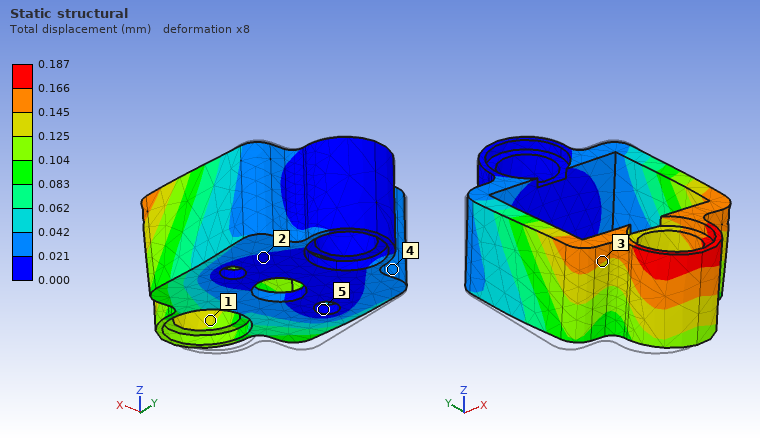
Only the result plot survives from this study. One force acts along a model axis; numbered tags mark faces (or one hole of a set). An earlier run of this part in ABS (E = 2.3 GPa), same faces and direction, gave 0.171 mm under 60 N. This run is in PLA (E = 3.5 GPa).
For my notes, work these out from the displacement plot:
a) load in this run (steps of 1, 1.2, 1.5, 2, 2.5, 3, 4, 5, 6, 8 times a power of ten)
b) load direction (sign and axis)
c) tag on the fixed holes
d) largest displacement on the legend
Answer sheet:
100 N
+X
5
0.187 mm
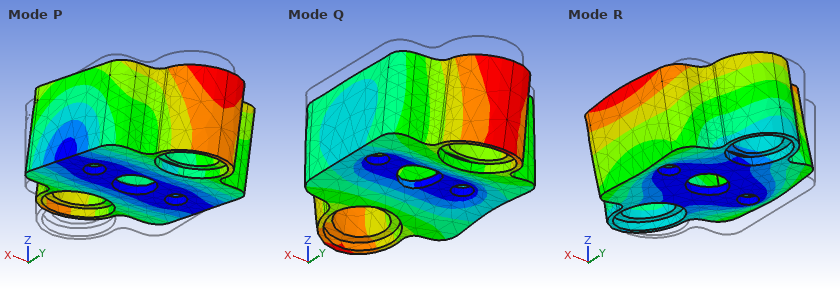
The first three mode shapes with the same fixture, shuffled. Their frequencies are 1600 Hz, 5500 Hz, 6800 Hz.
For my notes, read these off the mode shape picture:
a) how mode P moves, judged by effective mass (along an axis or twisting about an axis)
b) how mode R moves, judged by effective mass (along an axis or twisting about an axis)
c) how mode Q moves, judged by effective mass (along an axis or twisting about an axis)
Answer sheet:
along Y
along X
along Z
